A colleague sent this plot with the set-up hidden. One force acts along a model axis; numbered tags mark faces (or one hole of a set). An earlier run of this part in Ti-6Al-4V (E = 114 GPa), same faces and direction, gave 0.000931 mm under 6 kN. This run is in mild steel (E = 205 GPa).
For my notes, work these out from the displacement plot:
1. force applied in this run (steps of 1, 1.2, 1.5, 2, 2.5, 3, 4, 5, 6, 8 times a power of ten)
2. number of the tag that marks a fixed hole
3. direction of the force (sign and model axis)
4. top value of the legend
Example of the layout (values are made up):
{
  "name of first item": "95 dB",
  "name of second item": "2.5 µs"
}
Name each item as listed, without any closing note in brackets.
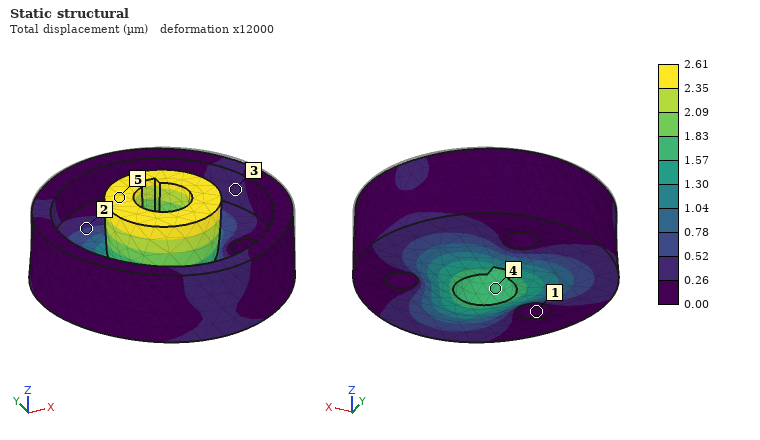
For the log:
{
  "force applied in this run": "30 kN",
  "number of the tag that marks a fixed hole": "1",
  "direction of the force": "-Z",
  "top value of the legend": "2.61 µm"
}
